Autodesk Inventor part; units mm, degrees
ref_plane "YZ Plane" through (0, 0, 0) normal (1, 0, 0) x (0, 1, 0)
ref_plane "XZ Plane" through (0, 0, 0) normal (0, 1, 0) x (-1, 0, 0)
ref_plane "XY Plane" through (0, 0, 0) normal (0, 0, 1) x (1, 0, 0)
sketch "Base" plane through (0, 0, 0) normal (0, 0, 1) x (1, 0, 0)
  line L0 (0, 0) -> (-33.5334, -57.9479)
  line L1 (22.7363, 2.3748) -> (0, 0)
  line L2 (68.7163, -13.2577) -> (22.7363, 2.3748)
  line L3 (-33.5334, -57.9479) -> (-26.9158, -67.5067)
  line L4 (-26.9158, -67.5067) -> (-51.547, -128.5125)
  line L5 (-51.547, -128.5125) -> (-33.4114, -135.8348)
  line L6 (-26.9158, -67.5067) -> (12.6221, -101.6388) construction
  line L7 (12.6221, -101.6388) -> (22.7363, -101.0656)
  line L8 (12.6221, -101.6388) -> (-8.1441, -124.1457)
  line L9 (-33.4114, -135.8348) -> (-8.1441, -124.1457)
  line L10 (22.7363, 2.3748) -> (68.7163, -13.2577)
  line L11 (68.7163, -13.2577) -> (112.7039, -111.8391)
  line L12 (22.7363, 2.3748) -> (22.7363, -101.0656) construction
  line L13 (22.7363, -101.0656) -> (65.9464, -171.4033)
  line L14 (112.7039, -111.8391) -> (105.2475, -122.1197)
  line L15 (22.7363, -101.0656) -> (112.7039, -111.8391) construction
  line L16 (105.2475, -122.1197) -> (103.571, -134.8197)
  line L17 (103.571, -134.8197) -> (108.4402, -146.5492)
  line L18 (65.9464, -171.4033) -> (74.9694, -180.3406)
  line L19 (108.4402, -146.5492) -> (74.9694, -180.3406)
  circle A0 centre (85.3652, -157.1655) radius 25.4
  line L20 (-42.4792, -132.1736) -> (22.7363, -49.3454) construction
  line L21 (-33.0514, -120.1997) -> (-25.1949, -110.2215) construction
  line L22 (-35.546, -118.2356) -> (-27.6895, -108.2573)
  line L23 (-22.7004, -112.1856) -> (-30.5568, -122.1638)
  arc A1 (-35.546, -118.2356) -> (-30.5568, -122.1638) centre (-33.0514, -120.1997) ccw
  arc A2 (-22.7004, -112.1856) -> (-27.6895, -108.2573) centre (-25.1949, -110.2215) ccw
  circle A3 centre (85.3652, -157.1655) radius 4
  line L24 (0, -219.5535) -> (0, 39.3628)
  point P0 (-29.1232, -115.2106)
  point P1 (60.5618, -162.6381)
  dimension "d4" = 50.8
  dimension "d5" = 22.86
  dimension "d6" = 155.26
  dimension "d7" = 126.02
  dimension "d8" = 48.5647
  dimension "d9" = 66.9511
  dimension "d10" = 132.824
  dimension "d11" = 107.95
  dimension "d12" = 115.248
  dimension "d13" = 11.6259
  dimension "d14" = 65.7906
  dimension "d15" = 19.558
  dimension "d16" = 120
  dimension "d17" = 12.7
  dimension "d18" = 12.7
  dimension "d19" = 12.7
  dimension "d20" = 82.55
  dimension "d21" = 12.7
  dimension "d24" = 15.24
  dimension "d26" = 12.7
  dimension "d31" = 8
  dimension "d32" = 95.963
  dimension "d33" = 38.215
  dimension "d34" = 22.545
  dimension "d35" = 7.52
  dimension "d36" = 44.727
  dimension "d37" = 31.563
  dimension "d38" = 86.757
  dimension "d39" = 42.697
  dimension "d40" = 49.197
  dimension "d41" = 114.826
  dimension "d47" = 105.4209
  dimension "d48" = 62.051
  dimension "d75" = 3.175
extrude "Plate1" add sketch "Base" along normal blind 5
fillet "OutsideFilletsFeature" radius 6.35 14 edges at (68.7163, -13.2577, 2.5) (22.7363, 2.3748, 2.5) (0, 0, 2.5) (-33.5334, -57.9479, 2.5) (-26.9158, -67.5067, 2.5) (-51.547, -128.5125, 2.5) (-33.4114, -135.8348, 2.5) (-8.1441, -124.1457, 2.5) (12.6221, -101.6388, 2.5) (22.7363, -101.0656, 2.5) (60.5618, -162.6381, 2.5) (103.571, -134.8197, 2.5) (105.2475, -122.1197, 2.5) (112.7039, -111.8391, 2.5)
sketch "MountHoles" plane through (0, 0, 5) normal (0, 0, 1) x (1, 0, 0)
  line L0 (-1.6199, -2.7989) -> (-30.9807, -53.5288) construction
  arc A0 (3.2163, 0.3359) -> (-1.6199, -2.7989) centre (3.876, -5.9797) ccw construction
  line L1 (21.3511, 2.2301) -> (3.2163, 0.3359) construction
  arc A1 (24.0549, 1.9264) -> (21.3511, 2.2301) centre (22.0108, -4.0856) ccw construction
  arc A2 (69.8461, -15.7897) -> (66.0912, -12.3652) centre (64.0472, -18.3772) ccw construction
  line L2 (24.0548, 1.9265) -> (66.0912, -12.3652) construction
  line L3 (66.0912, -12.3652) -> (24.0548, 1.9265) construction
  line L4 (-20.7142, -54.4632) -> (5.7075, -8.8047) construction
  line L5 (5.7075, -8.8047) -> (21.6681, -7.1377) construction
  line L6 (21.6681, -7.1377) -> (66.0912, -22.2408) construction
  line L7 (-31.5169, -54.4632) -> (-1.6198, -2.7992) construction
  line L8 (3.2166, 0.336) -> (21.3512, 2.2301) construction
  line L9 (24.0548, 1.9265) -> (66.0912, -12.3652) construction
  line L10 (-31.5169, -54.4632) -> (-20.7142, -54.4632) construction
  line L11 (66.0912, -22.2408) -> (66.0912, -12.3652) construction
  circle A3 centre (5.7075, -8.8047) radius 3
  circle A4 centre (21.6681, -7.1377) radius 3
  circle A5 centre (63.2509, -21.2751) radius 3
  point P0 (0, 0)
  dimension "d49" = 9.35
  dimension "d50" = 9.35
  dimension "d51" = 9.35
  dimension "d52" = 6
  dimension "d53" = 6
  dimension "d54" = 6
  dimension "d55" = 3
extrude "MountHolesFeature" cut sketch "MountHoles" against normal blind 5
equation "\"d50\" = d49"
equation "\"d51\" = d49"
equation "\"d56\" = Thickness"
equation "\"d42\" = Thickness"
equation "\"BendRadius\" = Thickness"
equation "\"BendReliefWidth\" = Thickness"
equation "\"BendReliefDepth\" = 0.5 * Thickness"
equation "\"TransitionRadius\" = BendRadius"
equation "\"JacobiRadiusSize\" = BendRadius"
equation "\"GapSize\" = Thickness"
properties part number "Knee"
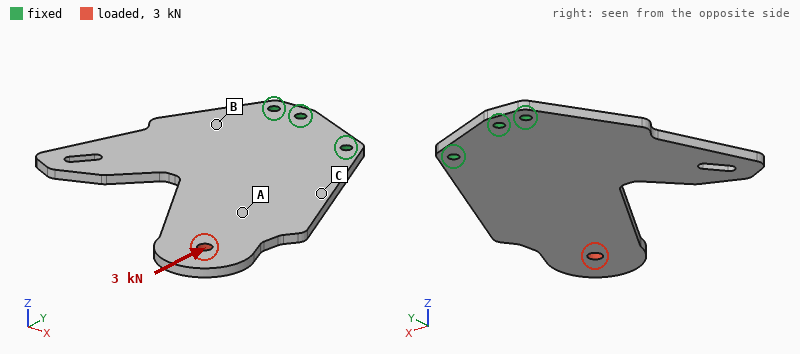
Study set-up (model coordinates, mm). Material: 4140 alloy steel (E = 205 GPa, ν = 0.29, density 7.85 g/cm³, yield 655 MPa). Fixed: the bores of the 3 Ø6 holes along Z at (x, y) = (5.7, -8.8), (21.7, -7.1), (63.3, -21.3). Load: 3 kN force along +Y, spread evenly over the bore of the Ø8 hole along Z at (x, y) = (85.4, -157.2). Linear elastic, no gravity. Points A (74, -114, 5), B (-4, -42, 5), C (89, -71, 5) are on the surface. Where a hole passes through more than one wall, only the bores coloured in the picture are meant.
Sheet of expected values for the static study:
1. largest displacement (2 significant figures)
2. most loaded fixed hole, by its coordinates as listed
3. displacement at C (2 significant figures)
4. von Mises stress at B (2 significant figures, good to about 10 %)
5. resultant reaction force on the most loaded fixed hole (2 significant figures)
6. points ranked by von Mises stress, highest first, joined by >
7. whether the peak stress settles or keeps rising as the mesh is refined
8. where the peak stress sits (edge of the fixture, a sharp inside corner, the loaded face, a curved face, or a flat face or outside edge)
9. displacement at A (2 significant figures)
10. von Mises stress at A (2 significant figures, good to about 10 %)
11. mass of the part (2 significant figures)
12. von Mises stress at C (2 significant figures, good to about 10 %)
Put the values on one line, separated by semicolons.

39 µm; (63.3, -21.3); 13 µm; 6.4 MPa; 3.9 kN; C > A > B; keeps rising; edge of the fixture; 18 µm; 13 MPa; 660 g; 20 MPa
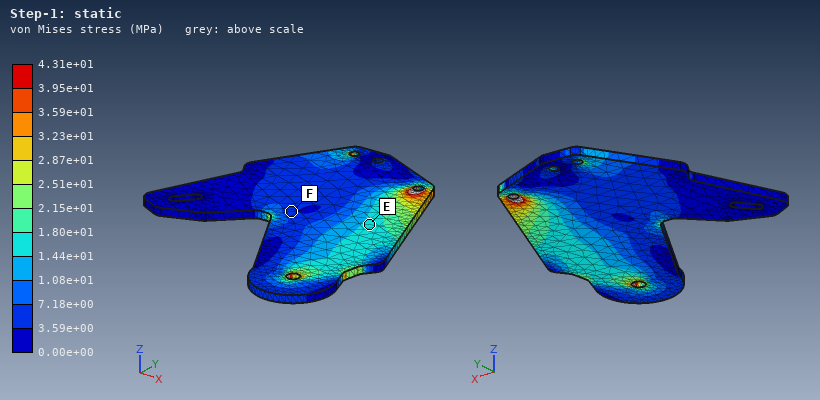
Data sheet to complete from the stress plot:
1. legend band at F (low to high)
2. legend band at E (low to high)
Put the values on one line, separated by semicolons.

3.59e+00 to 7.18e+00 MPa; 1.44e+01 to 1.80e+01 MPa
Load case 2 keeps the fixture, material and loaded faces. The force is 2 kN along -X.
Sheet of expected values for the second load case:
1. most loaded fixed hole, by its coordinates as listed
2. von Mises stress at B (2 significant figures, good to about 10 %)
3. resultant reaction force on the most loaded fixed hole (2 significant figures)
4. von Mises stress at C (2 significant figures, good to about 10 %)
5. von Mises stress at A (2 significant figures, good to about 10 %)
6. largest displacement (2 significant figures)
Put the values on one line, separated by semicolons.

(63.3, -21.3); 18 MPa; 5.0 kN; 20 MPa; 10 MPa; 72 µm
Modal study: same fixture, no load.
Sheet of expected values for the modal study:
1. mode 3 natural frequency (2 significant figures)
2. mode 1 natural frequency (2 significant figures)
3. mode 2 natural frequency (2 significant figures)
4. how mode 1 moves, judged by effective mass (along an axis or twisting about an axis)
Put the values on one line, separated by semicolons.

1000 Hz; 180 Hz; 390 Hz; along Z
